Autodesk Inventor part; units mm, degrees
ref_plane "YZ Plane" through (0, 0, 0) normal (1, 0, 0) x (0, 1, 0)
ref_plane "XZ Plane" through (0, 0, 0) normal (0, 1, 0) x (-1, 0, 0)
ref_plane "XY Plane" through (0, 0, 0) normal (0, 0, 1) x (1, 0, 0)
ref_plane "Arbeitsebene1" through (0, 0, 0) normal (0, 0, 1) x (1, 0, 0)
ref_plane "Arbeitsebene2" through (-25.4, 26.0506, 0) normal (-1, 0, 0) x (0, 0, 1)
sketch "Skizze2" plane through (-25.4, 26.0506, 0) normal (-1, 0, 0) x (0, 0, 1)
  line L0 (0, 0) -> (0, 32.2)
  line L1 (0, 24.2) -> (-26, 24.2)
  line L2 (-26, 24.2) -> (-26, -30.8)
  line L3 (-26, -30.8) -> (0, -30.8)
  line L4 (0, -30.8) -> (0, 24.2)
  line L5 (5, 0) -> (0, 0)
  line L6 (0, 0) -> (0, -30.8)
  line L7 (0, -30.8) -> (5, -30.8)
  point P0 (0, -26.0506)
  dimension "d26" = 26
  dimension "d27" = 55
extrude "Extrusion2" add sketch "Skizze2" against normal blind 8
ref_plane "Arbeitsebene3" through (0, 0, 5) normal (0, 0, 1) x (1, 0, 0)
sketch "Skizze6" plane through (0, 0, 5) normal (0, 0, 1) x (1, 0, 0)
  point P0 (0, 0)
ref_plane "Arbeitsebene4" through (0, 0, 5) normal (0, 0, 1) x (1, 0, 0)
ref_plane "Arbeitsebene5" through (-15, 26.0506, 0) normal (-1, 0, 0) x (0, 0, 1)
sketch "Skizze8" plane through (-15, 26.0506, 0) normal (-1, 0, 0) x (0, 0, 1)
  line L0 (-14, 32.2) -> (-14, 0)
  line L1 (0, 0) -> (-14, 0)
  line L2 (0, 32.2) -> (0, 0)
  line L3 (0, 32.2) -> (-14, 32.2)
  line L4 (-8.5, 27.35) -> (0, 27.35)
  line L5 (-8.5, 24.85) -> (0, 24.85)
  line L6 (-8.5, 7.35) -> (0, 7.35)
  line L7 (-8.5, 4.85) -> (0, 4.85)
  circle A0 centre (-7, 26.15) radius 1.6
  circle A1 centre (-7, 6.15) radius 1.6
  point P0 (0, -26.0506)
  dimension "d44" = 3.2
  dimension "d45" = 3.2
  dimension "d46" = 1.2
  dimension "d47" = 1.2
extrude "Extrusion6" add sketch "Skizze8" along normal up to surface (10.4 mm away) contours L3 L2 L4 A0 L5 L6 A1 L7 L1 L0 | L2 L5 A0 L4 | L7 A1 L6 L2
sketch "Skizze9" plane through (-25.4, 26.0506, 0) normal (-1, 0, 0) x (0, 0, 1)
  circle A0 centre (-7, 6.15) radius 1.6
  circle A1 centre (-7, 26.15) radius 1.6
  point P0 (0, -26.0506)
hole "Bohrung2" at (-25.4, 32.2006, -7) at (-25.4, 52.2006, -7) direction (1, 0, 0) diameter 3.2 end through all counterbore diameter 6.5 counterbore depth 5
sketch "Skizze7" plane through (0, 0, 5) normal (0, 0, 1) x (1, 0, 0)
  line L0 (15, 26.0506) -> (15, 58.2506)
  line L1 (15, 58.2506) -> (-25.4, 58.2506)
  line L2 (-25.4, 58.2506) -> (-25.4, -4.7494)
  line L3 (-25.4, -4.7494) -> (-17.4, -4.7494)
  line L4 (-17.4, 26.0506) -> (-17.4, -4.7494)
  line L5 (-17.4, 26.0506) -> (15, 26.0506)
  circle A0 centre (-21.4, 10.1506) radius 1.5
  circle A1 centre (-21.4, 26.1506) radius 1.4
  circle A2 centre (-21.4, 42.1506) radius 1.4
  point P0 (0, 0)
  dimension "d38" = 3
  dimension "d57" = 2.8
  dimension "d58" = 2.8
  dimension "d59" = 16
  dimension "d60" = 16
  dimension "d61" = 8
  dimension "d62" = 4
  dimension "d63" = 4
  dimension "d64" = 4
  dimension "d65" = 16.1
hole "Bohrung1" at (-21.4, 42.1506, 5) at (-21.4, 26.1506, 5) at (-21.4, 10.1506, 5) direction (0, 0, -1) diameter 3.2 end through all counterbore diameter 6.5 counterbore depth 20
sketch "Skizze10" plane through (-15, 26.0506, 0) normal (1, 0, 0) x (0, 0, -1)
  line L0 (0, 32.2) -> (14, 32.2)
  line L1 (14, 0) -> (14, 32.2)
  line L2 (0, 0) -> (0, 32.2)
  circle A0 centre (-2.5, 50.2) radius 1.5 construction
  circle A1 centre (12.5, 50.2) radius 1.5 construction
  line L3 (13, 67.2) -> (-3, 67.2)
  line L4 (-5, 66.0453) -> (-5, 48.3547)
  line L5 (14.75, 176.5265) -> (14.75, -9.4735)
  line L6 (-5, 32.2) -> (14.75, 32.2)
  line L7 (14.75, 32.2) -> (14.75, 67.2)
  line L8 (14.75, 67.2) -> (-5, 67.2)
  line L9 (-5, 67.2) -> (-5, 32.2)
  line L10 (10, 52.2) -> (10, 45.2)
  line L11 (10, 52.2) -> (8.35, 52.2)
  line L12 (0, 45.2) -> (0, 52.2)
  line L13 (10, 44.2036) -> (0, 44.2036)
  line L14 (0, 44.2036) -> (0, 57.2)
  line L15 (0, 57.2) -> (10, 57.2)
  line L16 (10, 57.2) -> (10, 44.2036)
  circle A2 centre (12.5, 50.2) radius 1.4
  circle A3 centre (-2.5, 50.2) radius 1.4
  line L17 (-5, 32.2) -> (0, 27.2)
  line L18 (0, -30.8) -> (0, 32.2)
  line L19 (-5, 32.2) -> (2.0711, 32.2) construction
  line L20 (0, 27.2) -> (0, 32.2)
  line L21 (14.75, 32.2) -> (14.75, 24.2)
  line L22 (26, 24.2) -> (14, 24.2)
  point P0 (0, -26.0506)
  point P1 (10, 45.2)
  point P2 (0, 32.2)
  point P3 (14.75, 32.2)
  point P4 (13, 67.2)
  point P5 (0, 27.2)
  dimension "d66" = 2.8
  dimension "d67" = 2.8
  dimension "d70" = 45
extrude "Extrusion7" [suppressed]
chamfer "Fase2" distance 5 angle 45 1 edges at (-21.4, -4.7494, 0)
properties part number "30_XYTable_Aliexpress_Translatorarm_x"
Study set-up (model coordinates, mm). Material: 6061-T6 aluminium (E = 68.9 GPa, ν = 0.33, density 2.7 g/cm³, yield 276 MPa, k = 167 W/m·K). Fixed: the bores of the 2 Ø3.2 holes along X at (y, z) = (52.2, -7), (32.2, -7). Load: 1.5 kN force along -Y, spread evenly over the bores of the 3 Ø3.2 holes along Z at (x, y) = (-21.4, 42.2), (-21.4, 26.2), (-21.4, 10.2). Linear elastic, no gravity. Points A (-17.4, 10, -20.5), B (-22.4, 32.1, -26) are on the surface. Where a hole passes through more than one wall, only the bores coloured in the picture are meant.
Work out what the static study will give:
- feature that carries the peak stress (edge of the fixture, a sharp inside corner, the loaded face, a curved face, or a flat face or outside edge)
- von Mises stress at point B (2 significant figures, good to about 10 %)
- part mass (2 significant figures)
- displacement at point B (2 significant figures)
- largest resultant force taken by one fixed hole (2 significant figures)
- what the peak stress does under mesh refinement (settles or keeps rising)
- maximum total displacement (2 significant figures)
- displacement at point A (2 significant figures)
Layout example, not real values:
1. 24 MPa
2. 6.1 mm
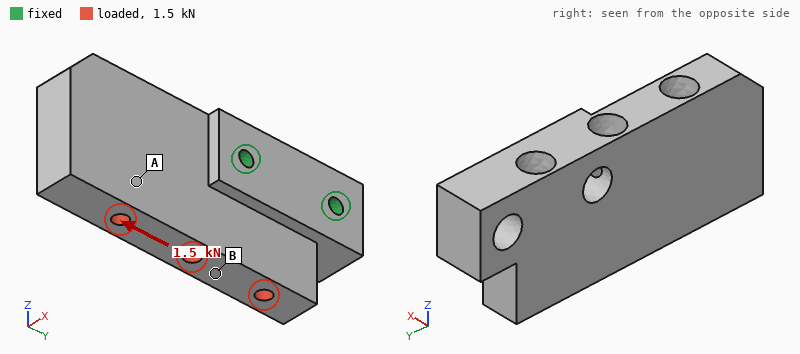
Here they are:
1. edge of the fixture
2. 12 MPa
3. 30 g
4. 12 µm
5. 1.2 kN
6. keeps rising
7. 30 µm
8. 18 µm
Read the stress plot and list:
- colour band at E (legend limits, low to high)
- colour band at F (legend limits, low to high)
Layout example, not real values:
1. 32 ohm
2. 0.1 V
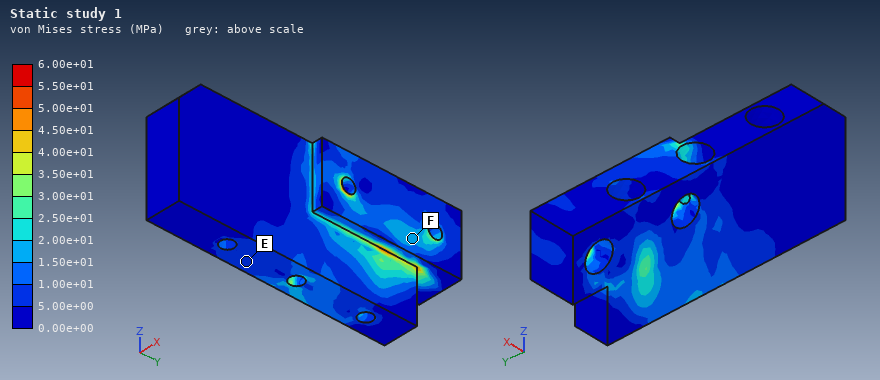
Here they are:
1. 5.00e+00 to 1.00e+01 MPa
2. 1.50e+01 to 2.00e+01 MPa
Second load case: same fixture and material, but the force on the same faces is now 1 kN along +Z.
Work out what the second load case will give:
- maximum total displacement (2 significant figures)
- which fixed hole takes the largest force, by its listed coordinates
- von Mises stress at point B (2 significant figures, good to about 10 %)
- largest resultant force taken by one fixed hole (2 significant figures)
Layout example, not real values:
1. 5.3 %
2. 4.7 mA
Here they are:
1. 35 µm
2. (32.2, -7)
3. 11 MPa
4. 1.2 kN
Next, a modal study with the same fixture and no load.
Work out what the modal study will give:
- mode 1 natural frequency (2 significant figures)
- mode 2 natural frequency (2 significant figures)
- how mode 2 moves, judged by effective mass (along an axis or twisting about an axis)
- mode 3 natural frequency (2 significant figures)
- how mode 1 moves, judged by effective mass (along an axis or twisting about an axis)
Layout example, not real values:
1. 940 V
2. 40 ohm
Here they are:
1. 3400 Hz
2. 6200 Hz
3. along Z
4. 7700 Hz
5. along X
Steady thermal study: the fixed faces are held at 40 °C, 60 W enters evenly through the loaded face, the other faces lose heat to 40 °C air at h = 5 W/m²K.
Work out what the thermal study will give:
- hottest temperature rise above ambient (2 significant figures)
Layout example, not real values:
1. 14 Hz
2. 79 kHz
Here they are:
1. 46 K
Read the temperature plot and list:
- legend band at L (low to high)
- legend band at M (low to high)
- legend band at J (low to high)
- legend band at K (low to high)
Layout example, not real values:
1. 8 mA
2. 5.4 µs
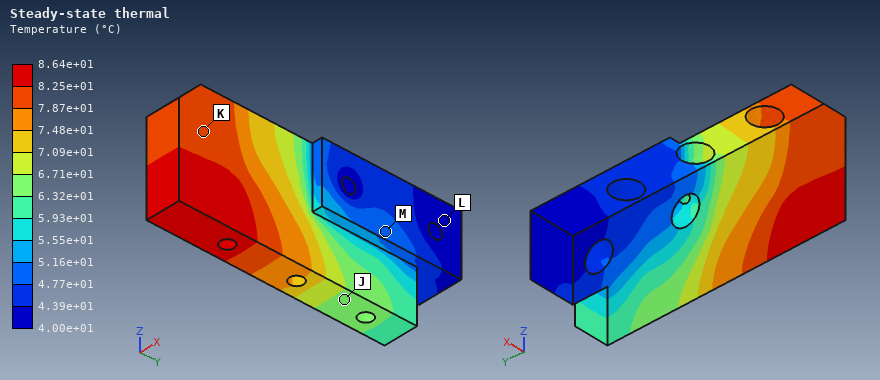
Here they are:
1. 4.00e+01 to 4.39e+01 °C
2. 4.77e+01 to 5.16e+01 °C
3. 6.32e+01 to 6.71e+01 °C
4. 7.87e+01 to 8.25e+01 °C
